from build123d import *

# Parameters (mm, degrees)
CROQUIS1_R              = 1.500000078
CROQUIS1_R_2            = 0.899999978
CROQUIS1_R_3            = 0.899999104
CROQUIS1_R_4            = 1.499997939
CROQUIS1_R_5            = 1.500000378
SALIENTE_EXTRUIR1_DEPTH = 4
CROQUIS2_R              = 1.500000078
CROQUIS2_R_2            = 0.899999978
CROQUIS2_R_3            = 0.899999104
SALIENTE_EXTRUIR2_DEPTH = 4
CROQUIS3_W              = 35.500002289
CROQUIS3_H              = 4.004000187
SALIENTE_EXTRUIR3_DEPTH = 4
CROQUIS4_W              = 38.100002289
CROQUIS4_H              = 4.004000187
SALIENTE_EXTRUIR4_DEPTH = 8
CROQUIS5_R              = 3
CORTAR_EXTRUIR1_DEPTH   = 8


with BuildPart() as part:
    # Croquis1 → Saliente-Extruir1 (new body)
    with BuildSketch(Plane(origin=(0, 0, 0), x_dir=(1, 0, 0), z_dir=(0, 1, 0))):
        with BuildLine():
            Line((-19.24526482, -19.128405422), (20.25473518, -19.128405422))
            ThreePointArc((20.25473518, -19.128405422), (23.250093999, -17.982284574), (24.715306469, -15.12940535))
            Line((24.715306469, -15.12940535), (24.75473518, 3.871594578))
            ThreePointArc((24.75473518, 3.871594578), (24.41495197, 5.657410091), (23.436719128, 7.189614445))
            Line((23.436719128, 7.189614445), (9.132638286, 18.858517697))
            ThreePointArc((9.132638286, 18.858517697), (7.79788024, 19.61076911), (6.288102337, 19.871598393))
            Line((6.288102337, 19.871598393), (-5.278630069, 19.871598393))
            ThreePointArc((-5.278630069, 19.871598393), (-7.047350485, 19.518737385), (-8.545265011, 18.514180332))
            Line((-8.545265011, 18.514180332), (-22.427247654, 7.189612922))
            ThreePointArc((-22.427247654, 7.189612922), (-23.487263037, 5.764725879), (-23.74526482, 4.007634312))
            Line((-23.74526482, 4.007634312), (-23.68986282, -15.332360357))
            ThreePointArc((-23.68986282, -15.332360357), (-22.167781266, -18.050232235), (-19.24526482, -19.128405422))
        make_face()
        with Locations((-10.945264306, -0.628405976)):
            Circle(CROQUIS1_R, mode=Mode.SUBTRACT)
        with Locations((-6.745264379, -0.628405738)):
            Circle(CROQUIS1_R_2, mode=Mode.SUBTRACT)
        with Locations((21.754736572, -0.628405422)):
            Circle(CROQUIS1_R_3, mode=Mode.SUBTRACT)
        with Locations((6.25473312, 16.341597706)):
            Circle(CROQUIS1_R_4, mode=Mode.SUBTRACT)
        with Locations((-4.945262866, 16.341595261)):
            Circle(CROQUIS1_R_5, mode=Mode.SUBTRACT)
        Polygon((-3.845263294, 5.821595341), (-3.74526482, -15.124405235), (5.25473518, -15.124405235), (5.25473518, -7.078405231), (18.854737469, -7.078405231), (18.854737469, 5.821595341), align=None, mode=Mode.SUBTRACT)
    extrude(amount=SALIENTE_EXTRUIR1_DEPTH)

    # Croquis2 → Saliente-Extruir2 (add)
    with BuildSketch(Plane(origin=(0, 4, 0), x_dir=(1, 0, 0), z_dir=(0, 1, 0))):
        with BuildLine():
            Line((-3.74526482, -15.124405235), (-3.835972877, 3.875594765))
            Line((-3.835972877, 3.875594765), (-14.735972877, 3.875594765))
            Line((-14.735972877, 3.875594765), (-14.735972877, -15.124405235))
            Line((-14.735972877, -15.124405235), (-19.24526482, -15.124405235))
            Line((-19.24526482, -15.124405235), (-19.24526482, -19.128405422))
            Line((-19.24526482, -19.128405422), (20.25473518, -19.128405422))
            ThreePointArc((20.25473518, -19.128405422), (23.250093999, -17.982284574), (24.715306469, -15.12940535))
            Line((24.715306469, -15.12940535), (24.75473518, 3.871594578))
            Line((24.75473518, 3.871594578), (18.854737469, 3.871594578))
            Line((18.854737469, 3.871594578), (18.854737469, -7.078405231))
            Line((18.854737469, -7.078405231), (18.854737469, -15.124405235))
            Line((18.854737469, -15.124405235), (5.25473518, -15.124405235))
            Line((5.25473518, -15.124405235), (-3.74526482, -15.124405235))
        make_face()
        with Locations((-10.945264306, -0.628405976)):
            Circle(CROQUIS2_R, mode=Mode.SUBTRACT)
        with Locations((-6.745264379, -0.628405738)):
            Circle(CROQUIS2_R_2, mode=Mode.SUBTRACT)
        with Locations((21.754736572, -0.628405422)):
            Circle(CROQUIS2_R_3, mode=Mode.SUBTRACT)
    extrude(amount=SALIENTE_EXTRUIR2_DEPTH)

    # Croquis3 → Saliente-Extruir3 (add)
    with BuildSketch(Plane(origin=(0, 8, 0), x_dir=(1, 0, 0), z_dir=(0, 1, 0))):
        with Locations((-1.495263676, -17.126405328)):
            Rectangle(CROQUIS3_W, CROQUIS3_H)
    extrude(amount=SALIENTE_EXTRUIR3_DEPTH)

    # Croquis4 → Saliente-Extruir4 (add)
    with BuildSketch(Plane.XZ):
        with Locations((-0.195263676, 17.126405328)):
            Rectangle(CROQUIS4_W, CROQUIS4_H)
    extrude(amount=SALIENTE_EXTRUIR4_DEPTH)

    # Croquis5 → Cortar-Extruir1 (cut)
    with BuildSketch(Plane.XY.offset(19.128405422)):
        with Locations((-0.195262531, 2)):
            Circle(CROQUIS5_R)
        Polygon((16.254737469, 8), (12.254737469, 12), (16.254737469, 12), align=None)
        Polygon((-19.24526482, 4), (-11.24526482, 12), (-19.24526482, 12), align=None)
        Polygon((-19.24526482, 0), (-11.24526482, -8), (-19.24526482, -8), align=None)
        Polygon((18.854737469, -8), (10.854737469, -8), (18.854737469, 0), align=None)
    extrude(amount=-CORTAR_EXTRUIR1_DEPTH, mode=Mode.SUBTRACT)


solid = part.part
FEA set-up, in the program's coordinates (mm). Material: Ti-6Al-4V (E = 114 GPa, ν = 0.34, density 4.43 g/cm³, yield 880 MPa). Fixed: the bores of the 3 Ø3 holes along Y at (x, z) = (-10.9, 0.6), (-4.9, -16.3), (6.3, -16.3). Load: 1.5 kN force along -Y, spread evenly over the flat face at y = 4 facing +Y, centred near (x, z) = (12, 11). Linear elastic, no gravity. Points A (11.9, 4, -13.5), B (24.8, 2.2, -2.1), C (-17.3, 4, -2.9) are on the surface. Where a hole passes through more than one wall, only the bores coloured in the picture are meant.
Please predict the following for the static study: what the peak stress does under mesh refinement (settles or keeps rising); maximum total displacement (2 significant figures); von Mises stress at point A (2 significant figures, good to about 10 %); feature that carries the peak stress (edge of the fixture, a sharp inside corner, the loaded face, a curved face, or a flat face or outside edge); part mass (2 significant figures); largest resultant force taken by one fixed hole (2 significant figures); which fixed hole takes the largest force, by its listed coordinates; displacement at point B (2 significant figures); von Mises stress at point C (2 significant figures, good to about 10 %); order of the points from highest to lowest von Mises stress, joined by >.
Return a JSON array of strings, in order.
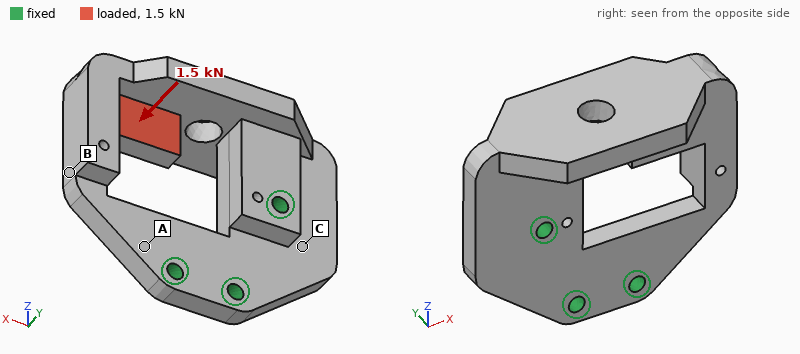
["keeps rising", "0.28 mm", "160 MPa", "edge of the fixture", "36 g", "1.2 kN", "(-10.9, 0.6)", "0.17 mm", "58 MPa", "A > C > B"]
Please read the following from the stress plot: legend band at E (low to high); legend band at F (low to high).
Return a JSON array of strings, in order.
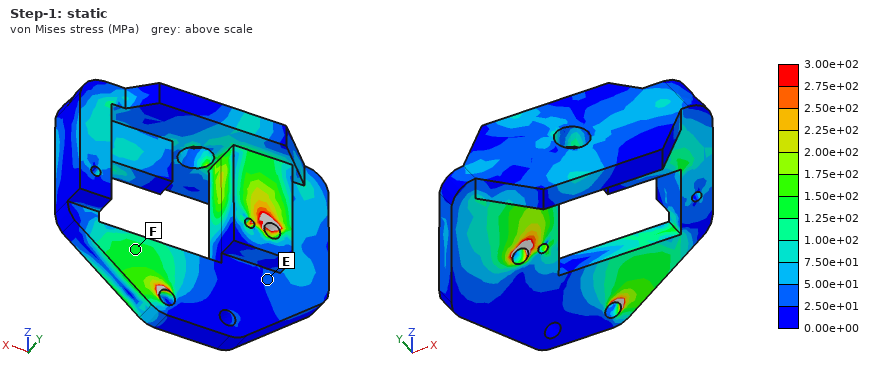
["2.50e+01 to 5.00e+01 MPa", "1.25e+02 to 1.50e+02 MPa"]
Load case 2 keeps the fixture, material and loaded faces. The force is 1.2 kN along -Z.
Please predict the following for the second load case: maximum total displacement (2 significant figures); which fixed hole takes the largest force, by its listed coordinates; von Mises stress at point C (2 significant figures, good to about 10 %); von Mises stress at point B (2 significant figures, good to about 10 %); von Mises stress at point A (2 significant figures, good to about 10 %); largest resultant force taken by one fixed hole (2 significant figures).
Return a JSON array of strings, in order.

["37 µm", "(6.3, -16.3)", "16 MPa", "27 MPa", "43 MPa", "1.1 kN"]
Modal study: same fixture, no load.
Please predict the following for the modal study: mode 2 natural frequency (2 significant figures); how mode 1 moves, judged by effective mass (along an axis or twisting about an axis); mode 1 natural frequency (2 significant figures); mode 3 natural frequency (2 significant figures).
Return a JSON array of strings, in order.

["7700 Hz", "along Y", "3600 Hz", "8500 Hz"]
